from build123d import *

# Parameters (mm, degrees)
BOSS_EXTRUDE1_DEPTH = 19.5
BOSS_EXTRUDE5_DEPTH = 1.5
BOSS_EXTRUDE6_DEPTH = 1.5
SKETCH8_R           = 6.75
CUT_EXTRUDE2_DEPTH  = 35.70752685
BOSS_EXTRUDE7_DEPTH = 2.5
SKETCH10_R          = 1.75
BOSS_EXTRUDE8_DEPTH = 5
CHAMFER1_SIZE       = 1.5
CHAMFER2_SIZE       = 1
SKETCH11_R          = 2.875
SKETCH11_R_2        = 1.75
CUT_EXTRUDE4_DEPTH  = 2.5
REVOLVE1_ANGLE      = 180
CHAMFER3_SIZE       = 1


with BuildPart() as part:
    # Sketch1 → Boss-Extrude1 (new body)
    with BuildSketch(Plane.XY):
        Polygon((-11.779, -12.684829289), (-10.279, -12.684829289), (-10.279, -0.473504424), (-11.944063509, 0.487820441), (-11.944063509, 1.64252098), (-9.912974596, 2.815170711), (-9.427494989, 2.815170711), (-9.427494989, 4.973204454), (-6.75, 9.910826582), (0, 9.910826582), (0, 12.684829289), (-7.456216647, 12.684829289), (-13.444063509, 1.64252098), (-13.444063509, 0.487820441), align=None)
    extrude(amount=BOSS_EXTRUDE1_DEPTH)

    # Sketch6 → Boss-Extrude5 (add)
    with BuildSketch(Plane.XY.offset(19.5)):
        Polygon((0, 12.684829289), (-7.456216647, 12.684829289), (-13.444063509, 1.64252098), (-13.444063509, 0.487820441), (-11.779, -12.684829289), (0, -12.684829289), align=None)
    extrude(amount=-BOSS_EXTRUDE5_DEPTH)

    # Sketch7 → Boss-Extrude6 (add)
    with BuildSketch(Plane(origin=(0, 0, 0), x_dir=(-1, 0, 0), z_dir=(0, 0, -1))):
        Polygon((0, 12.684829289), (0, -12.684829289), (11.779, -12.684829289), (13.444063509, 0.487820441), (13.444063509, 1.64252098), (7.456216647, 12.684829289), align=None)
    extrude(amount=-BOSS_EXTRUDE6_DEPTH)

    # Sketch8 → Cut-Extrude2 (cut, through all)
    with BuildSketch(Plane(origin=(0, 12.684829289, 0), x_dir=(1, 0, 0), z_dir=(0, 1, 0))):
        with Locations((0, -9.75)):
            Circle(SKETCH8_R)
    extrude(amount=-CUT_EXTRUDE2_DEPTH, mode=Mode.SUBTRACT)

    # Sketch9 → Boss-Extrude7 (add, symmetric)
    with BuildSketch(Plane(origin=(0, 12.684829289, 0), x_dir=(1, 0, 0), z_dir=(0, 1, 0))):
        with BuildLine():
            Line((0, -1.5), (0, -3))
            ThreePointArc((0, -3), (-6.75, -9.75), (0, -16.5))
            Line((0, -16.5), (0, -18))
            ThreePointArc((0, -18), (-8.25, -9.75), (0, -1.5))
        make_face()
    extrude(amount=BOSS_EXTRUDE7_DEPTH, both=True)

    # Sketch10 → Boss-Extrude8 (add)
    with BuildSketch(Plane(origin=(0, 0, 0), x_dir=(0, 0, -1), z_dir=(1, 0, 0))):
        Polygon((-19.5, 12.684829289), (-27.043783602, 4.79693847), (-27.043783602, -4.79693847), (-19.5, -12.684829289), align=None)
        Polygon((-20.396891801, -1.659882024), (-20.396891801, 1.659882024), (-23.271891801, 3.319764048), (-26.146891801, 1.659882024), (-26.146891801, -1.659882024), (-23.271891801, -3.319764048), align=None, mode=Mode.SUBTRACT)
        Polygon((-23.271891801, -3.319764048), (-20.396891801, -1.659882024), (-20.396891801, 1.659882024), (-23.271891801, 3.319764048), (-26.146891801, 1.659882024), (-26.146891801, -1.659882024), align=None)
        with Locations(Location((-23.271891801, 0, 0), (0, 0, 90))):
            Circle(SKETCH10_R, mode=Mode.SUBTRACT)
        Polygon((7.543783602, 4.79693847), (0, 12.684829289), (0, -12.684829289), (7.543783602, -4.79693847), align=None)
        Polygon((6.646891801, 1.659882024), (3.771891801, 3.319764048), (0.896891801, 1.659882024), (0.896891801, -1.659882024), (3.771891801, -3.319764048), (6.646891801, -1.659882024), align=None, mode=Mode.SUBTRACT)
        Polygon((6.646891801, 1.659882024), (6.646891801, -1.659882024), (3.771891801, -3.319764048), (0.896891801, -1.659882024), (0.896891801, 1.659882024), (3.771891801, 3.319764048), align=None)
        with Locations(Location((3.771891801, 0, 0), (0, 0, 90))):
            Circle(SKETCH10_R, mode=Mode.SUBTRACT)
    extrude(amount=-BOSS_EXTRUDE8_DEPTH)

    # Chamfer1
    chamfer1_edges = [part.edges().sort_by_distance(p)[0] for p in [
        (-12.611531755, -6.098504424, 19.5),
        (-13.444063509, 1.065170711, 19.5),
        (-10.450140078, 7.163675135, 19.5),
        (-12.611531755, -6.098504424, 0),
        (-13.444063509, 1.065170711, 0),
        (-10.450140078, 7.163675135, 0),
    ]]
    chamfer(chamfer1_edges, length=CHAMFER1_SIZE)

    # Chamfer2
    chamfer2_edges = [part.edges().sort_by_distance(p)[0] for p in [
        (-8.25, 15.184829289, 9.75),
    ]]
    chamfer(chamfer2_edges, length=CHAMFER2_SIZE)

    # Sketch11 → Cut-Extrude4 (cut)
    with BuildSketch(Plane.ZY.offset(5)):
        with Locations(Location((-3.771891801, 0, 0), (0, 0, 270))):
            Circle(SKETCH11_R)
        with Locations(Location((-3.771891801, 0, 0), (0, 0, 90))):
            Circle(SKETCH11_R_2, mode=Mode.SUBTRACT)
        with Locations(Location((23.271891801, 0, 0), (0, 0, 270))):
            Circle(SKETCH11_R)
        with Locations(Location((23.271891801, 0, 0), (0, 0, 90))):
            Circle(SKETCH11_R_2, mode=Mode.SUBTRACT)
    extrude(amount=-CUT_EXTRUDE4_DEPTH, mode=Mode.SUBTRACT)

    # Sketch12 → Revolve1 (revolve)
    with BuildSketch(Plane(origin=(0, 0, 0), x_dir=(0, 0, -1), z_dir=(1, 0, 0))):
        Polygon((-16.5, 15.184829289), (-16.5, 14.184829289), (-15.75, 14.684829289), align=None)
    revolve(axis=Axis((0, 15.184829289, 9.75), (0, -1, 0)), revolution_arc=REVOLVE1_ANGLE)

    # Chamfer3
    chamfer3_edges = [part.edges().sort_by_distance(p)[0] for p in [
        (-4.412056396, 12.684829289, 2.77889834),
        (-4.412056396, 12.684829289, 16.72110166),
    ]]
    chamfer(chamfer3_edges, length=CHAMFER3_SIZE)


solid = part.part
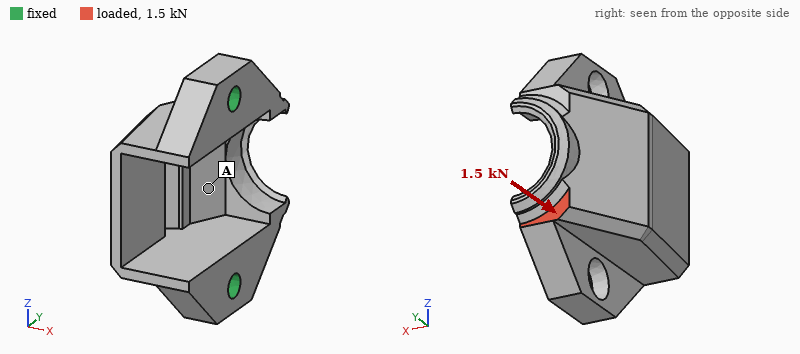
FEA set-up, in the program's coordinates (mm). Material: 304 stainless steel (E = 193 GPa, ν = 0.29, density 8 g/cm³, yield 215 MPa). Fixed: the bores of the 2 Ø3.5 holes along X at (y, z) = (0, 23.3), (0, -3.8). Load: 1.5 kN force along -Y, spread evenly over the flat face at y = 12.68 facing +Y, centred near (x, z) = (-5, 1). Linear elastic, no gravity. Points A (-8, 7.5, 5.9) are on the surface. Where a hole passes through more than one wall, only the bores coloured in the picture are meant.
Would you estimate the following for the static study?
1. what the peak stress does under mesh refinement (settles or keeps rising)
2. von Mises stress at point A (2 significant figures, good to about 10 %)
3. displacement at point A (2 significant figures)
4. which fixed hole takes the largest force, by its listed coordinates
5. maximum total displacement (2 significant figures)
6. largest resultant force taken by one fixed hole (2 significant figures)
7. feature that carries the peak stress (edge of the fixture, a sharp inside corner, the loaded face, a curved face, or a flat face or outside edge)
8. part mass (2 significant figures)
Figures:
keeps rising
29 MPa
13 µm
(0, -3.8)
20 µm
1.3 kN
edge of the fixture
25 g
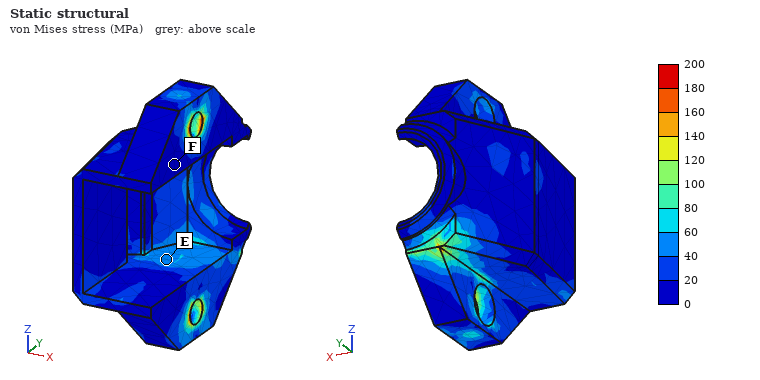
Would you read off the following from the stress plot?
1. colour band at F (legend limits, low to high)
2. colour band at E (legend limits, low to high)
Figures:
0 to 20 MPa
40 to 60 MPa
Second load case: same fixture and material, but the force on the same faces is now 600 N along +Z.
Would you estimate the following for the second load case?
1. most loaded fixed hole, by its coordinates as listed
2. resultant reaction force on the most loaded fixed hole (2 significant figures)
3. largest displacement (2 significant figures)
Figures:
(0, -3.8)
410 N
15 µm
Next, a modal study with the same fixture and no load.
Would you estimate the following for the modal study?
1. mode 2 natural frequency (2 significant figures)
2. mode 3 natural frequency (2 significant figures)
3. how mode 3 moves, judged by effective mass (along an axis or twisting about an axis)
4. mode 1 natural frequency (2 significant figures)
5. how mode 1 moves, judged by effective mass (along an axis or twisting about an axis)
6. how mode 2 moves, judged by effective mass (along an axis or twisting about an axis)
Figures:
13 kHz
17 kHz
along Z
8300 Hz
along Y
along Z
